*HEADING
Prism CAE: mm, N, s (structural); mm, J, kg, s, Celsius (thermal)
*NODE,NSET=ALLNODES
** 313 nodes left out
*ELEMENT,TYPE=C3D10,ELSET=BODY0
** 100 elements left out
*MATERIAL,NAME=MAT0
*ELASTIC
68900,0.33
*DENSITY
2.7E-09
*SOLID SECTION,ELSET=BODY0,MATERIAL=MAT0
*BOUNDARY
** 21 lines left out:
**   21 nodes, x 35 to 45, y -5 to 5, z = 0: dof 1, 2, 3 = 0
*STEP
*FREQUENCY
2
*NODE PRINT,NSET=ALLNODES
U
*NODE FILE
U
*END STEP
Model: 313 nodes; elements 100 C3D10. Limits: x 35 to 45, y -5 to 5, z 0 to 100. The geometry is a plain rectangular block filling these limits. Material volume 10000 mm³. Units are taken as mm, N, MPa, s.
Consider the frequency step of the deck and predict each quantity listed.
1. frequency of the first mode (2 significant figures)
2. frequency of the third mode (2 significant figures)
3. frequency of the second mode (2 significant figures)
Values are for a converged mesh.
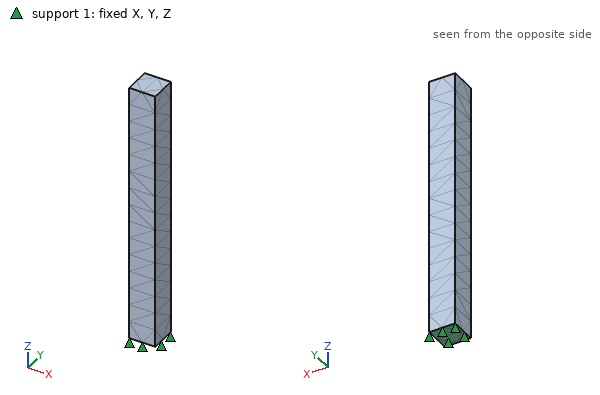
820 Hz
4900 Hz
820 Hz
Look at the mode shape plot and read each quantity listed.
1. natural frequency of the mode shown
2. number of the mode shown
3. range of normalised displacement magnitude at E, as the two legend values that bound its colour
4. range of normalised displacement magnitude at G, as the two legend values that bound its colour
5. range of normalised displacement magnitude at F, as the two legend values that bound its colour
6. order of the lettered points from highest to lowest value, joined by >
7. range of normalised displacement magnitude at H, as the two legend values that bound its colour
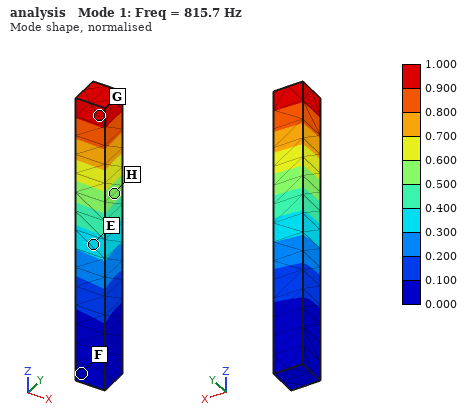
815.7 Hz
1
0.300 to 0.400
0.900 to 1.000
0.000 to 0.100
G > H > E > F
0.500 to 0.600
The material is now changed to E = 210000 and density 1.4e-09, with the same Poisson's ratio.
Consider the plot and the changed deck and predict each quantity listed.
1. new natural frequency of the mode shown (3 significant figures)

1980 Hz
